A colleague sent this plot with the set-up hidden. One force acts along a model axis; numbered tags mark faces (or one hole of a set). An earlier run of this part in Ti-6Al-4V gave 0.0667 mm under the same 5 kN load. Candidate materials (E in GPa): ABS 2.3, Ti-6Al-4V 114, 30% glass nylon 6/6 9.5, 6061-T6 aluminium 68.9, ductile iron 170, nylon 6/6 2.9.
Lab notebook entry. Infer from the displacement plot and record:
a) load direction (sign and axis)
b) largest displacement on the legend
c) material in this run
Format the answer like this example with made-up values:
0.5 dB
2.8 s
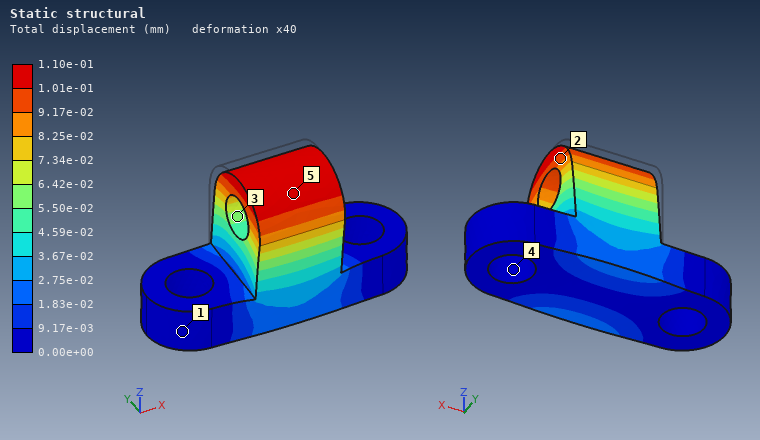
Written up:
-Y
1.10e-01 mm
6061-T6 aluminium
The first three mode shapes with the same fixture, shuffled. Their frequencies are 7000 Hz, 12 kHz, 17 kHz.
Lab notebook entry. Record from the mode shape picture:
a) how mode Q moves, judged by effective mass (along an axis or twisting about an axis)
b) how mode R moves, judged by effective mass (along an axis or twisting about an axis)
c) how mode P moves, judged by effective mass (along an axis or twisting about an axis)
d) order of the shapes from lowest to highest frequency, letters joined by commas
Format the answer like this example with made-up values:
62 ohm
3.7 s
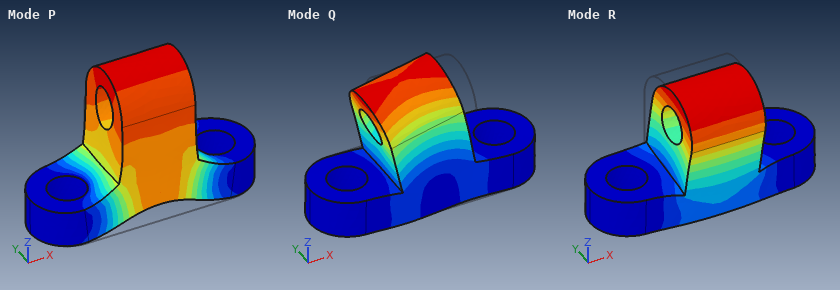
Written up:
along X
along Y
along Z
R, Q, P
